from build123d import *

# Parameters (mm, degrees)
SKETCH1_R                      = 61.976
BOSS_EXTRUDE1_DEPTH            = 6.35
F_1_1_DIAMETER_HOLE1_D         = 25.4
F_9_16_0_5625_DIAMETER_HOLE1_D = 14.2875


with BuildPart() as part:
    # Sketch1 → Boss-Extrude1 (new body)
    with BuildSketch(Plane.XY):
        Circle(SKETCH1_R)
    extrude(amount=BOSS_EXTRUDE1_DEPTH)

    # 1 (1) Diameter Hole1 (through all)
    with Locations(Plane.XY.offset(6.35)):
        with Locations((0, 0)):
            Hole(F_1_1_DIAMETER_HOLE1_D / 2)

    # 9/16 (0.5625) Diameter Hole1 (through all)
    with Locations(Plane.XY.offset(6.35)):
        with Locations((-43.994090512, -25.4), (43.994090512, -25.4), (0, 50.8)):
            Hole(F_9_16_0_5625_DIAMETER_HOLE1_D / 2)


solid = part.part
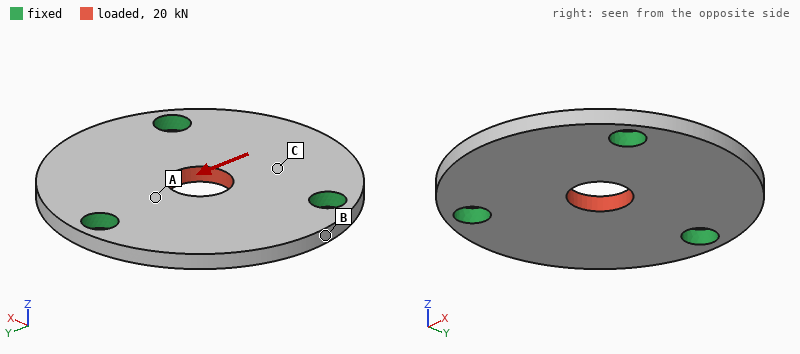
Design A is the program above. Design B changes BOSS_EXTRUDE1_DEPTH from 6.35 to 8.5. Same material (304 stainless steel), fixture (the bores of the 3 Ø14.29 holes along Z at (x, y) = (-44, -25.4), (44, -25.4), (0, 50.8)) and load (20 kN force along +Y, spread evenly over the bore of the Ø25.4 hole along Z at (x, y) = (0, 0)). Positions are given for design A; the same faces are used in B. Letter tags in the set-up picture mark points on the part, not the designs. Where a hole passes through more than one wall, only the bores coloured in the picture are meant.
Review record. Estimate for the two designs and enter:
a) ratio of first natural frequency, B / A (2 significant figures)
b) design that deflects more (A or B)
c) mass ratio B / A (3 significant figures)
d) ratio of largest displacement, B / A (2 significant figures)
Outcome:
1.3
A
1.34
0.75
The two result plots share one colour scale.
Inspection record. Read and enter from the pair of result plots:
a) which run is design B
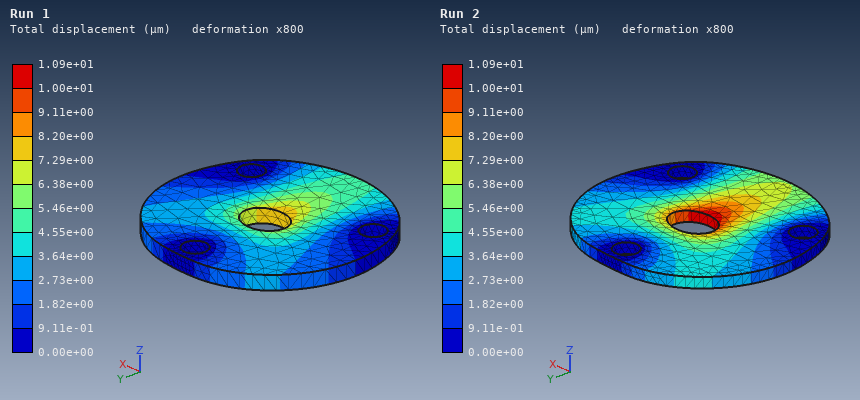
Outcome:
Run 1
